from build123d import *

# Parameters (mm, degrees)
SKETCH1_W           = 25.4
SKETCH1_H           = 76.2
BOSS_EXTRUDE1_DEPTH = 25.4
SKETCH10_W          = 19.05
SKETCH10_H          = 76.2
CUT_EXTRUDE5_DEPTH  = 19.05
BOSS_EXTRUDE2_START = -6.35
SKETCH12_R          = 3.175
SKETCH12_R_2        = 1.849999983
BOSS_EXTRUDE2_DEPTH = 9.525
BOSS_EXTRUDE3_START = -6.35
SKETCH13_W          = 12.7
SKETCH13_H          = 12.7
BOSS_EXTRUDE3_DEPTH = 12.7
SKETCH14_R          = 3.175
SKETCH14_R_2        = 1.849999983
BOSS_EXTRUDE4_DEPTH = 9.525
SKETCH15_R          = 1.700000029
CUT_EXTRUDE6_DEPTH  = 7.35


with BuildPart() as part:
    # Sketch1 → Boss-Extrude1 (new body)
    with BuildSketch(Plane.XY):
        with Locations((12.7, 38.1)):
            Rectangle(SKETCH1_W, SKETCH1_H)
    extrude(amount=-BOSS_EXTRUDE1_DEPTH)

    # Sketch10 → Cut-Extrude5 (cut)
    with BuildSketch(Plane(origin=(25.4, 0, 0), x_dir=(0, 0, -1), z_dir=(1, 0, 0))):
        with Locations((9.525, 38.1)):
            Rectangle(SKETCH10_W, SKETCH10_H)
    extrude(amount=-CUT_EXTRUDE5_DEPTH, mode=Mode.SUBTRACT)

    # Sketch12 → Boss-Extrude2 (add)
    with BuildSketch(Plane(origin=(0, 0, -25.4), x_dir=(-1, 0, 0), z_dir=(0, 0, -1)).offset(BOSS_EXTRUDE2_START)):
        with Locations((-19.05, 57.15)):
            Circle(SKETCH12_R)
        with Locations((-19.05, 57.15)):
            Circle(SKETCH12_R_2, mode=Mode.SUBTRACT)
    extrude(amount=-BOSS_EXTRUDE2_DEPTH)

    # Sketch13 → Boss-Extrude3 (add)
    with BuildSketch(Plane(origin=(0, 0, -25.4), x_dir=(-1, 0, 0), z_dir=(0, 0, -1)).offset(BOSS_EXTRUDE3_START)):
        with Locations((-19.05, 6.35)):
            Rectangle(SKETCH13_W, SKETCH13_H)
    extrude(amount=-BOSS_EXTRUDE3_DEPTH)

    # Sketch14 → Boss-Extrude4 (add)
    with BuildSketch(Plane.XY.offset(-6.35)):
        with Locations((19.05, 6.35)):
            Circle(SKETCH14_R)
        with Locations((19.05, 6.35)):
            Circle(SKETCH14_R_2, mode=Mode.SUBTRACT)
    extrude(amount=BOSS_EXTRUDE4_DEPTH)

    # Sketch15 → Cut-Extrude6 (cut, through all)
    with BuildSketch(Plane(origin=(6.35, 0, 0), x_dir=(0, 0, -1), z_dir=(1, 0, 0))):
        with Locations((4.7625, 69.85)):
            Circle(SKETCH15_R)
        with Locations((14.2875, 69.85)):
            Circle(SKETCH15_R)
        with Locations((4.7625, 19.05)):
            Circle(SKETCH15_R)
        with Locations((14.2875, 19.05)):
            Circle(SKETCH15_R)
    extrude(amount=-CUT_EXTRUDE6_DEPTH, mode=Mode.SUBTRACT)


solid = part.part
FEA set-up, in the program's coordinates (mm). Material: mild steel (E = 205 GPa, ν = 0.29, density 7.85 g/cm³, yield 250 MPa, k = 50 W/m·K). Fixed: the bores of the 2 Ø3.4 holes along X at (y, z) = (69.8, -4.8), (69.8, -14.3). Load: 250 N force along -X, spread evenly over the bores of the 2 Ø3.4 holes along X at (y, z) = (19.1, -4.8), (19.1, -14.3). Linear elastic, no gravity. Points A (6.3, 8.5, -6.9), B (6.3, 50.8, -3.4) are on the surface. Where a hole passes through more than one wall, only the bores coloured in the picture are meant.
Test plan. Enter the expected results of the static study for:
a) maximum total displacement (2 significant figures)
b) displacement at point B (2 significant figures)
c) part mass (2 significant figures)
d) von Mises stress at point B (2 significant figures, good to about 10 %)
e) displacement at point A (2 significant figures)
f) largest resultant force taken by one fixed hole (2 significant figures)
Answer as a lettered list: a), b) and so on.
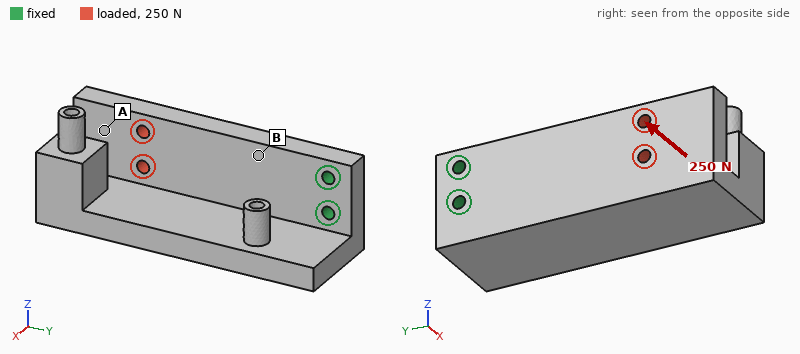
a) 60 µm
b) 11 µm
c) 190 g
d) 15 MPa
e) 52 µm
f) 130 N
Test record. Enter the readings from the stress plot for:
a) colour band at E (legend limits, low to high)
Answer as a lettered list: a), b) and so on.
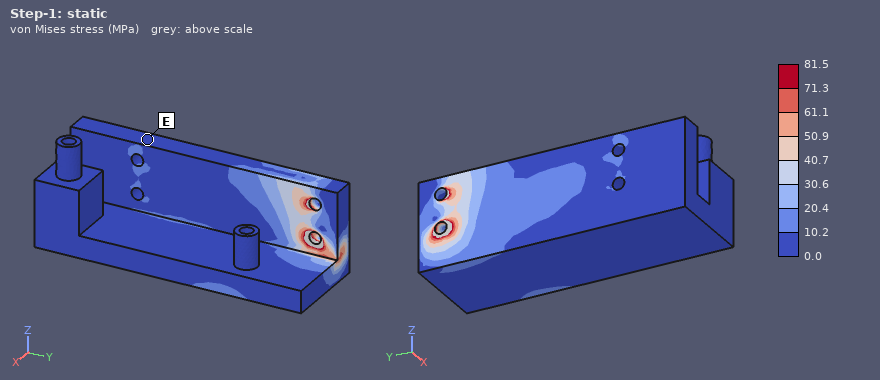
a) 0.0 to 10.2 MPa
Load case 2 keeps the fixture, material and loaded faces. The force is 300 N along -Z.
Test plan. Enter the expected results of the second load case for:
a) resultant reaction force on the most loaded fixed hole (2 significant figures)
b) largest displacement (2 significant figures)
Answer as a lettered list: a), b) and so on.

a) 1.2 kN
b) 18 µm
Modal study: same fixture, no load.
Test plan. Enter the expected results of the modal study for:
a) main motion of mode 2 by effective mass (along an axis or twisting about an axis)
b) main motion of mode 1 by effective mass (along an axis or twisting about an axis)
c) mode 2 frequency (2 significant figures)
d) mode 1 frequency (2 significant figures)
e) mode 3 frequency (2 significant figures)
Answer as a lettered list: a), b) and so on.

a) along Z
b) along X
c) 1900 Hz
d) 1100 Hz
e) 3500 Hz
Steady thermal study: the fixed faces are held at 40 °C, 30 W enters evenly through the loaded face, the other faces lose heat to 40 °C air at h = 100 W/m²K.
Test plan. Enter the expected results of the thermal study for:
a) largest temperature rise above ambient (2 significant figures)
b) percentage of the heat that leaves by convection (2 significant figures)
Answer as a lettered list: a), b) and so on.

a) 68 K
b) 76 %
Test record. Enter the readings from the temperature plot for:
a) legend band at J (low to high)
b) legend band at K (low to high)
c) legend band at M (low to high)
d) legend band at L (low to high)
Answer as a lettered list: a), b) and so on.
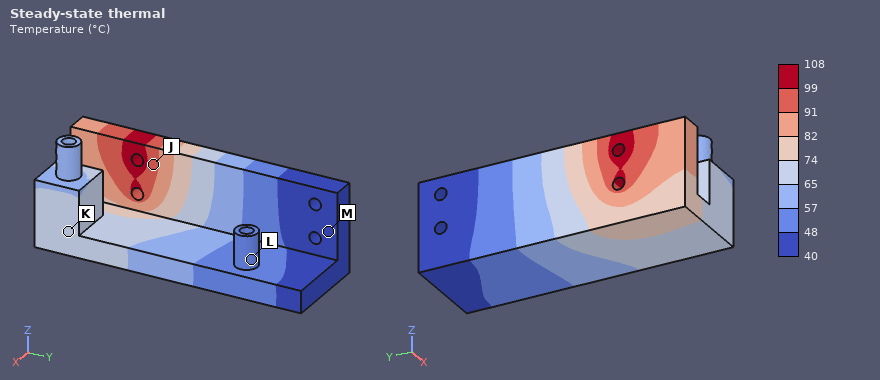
a) 91 to 99 °C
b) 65 to 74 °C
c) 40 to 48 °C
d) 48 to 57 °C
